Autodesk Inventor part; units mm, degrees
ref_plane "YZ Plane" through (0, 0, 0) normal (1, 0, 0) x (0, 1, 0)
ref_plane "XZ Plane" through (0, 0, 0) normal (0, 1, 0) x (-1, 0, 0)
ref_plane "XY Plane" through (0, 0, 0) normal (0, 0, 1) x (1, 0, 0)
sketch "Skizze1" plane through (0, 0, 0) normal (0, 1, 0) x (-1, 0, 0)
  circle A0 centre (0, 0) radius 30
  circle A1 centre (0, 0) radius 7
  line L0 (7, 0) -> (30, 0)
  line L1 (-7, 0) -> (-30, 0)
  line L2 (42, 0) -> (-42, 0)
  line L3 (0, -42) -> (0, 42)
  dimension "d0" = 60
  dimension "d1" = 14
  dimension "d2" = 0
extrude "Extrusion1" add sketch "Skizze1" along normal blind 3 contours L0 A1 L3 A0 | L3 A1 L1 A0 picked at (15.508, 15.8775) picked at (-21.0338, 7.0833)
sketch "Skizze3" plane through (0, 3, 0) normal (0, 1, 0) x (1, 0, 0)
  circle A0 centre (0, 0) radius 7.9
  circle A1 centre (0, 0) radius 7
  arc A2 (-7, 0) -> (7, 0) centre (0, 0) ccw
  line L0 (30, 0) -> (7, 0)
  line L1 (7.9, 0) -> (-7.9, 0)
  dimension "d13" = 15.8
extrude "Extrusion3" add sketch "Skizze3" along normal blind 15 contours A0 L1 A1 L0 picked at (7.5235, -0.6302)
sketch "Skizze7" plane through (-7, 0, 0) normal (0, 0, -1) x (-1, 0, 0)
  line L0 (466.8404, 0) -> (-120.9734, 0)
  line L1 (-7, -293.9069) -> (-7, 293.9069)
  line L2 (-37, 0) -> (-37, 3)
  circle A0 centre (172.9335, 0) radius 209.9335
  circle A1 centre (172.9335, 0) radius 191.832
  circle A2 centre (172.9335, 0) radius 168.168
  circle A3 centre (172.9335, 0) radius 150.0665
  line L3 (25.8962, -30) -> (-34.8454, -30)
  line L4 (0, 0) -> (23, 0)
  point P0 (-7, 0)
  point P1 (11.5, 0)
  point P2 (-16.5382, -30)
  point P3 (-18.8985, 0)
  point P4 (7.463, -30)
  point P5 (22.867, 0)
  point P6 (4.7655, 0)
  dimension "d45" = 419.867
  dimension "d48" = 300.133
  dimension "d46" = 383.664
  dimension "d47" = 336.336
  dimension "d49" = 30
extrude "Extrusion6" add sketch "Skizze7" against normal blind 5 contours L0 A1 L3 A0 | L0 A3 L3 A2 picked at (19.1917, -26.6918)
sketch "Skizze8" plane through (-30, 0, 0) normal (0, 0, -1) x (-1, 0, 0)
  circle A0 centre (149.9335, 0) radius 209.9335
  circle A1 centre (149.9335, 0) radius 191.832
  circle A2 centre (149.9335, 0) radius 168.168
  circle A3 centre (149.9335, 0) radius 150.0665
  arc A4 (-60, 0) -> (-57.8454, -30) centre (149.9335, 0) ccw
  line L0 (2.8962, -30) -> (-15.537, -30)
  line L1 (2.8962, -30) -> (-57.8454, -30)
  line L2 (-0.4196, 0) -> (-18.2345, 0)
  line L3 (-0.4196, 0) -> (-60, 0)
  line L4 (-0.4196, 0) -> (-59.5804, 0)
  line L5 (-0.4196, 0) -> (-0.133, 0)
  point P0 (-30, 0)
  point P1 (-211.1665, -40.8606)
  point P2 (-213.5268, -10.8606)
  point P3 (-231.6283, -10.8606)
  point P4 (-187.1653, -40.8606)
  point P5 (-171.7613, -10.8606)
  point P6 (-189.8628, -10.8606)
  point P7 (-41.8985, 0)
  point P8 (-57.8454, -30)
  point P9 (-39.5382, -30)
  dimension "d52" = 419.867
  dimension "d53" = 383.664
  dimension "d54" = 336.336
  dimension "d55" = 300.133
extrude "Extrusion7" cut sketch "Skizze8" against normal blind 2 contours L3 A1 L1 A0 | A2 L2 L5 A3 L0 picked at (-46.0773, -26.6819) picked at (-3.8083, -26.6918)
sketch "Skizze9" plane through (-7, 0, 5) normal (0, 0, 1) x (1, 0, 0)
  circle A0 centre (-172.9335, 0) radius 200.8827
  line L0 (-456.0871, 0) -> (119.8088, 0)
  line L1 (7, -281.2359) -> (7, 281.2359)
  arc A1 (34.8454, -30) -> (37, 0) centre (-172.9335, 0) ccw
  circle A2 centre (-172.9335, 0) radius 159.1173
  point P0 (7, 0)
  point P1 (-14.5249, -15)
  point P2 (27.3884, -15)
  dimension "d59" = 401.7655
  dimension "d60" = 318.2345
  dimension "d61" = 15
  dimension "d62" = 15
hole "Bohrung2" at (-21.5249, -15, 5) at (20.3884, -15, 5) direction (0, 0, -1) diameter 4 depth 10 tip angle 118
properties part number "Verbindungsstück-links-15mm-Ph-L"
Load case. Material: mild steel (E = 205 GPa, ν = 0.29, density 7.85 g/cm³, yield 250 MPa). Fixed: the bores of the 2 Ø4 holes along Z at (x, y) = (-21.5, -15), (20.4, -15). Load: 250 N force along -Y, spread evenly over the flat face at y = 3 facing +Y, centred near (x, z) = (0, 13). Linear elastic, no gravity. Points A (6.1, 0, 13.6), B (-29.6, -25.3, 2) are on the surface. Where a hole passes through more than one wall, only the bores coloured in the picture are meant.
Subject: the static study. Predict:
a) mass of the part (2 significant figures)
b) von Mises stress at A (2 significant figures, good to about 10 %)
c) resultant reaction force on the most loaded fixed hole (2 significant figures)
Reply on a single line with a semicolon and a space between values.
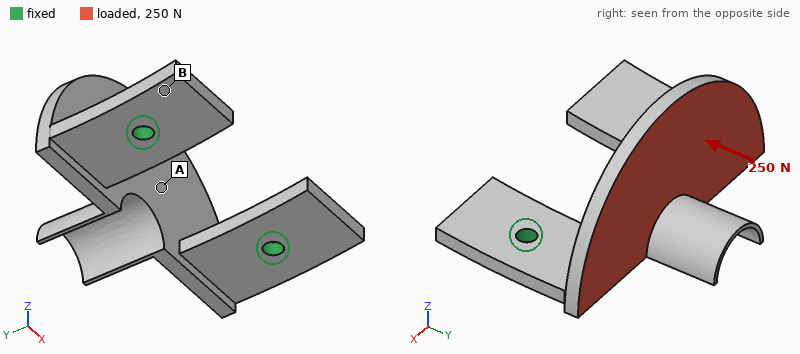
59 g; 9.8 MPa; 130 N
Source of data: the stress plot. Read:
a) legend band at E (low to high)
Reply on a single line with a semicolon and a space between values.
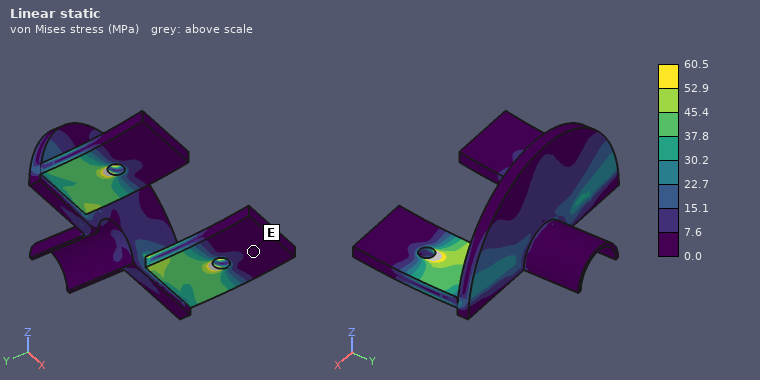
0.0 to 7.6 MPa
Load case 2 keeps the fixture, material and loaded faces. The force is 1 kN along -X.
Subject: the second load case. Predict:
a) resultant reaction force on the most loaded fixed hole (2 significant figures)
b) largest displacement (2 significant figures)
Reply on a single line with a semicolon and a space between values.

560 N; 35 µm
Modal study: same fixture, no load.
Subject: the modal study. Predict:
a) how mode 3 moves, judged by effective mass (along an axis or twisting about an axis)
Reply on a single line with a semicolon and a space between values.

along Z
